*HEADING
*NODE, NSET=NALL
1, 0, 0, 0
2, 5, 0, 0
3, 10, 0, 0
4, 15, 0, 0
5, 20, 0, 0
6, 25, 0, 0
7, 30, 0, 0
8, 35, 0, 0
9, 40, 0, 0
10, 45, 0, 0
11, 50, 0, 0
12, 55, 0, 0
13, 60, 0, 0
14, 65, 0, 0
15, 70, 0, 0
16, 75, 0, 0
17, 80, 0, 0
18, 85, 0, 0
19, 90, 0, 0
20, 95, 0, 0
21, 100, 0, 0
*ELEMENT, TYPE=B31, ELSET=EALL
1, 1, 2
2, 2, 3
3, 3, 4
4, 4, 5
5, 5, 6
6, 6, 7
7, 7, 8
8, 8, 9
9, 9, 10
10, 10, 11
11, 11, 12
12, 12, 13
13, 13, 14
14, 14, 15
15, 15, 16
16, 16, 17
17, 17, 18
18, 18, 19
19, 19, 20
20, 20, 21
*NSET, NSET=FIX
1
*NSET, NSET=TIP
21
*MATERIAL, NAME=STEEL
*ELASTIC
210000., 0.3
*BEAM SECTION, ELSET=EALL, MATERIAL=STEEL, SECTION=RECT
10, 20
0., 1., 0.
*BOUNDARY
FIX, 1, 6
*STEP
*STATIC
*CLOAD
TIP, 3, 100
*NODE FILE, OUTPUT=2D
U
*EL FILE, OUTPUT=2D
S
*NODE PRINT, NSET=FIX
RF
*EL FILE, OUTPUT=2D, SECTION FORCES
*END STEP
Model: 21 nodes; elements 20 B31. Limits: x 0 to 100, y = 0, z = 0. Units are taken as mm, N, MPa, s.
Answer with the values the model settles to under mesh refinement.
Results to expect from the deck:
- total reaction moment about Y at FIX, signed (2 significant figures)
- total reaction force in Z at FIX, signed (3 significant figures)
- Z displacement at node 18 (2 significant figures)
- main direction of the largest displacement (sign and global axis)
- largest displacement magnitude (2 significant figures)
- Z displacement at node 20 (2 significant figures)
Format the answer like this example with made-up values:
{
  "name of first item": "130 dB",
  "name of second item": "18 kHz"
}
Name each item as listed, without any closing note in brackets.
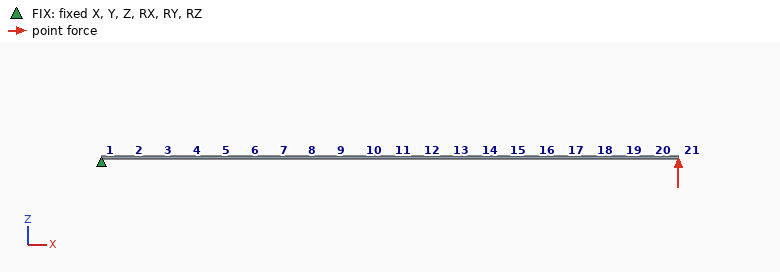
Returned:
{
  "total reaction moment about Y at FIX, signed": "10000 N·mm",
  "total reaction force in Z at FIX, signed": "-100 N",
  "Z displacement at node 18": "0.019 mm",
  "main direction of the largest displacement": "+Z",
  "largest displacement magnitude": "0.025 mm",
  "Z displacement at node 20": "0.023 mm"
}
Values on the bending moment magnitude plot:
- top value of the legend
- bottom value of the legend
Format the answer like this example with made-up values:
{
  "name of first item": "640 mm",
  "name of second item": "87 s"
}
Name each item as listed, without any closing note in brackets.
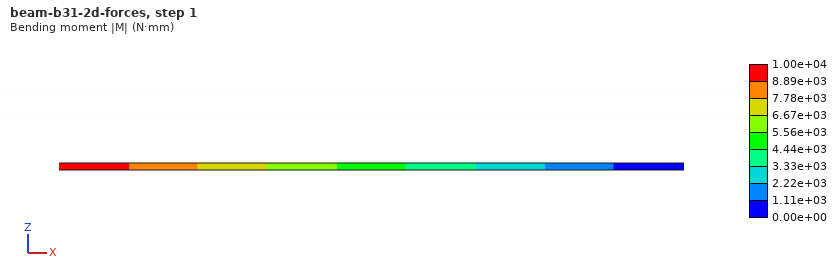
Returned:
{
  "top value of the legend": "1.00e+04 N·mm",
  "bottom value of the legend": "0.00e+00 N·mm"
}
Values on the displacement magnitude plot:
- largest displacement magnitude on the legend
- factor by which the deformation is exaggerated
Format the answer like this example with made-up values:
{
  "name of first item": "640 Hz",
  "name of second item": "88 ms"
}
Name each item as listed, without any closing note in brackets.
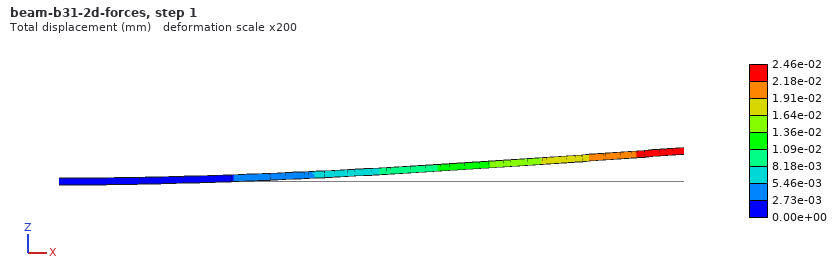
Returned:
{
  "largest displacement magnitude on the legend": "2.46e-02 mm",
  "factor by which the deformation is exaggerated": "200"
}
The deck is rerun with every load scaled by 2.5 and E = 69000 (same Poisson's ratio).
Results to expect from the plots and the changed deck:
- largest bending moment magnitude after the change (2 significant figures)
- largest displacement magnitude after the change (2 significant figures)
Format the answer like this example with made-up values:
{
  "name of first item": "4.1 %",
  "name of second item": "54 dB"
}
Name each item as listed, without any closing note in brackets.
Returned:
{
  "largest bending moment magnitude after the change": "25000 N·mm",
  "largest displacement magnitude after the change": "0.19 mm"
}
